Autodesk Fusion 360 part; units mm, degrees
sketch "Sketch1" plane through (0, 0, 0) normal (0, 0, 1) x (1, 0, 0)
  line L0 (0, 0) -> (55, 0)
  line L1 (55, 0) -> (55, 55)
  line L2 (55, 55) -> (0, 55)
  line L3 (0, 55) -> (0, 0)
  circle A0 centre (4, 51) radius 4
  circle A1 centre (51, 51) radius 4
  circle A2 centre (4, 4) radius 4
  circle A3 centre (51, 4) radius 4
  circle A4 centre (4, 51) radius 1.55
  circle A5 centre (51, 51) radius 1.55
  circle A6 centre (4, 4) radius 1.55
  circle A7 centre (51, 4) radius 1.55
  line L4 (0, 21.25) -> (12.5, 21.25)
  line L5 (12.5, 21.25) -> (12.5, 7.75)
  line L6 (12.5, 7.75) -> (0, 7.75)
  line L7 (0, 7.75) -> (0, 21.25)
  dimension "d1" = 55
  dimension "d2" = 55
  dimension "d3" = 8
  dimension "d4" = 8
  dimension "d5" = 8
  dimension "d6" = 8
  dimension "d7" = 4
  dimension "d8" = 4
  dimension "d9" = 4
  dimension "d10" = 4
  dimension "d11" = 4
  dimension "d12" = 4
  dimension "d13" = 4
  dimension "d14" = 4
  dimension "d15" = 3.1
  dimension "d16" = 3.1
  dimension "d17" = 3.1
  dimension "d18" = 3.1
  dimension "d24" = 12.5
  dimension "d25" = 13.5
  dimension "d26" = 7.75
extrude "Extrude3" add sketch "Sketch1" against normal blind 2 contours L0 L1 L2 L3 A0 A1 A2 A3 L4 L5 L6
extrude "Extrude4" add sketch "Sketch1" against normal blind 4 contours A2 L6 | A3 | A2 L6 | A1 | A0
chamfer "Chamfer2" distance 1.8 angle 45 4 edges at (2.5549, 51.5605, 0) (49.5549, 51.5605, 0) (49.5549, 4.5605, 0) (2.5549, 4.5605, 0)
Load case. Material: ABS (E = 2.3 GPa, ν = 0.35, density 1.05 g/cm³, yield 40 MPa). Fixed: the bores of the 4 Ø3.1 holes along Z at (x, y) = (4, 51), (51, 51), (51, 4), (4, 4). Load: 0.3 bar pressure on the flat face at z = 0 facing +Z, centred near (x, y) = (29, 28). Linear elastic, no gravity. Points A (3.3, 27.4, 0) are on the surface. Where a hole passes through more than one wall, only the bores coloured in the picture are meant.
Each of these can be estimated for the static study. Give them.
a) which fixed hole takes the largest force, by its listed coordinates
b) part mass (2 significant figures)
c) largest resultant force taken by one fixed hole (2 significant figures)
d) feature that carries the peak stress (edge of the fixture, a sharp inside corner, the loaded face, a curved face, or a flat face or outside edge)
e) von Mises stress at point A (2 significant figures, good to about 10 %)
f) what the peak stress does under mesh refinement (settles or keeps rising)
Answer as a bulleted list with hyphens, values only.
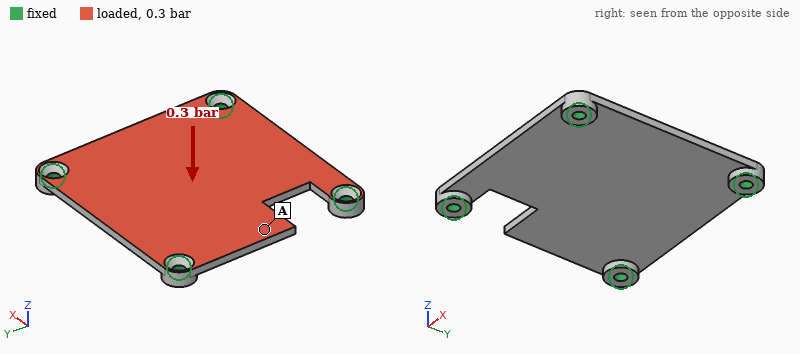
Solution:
- (51, 4)
- 6.2 g
- 44 N
- edge of the fixture
- 3.4 MPa
- keeps rising
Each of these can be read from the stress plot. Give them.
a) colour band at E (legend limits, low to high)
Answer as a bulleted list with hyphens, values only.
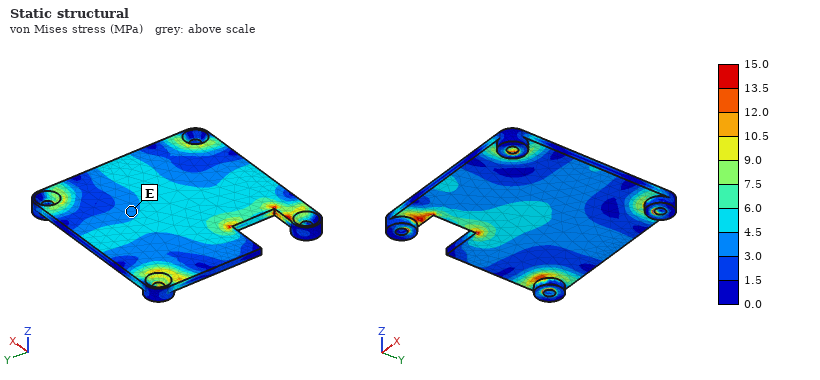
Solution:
- 3.0 to 4.5 MPa
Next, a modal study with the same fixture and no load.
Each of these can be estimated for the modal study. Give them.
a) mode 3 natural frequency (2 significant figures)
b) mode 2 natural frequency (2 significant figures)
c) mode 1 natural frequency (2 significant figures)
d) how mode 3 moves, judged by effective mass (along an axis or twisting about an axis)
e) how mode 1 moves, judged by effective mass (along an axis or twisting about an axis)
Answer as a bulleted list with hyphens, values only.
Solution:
- 1700 Hz
- 1400 Hz
- 910 Hz
- twisting about X
- along Z
